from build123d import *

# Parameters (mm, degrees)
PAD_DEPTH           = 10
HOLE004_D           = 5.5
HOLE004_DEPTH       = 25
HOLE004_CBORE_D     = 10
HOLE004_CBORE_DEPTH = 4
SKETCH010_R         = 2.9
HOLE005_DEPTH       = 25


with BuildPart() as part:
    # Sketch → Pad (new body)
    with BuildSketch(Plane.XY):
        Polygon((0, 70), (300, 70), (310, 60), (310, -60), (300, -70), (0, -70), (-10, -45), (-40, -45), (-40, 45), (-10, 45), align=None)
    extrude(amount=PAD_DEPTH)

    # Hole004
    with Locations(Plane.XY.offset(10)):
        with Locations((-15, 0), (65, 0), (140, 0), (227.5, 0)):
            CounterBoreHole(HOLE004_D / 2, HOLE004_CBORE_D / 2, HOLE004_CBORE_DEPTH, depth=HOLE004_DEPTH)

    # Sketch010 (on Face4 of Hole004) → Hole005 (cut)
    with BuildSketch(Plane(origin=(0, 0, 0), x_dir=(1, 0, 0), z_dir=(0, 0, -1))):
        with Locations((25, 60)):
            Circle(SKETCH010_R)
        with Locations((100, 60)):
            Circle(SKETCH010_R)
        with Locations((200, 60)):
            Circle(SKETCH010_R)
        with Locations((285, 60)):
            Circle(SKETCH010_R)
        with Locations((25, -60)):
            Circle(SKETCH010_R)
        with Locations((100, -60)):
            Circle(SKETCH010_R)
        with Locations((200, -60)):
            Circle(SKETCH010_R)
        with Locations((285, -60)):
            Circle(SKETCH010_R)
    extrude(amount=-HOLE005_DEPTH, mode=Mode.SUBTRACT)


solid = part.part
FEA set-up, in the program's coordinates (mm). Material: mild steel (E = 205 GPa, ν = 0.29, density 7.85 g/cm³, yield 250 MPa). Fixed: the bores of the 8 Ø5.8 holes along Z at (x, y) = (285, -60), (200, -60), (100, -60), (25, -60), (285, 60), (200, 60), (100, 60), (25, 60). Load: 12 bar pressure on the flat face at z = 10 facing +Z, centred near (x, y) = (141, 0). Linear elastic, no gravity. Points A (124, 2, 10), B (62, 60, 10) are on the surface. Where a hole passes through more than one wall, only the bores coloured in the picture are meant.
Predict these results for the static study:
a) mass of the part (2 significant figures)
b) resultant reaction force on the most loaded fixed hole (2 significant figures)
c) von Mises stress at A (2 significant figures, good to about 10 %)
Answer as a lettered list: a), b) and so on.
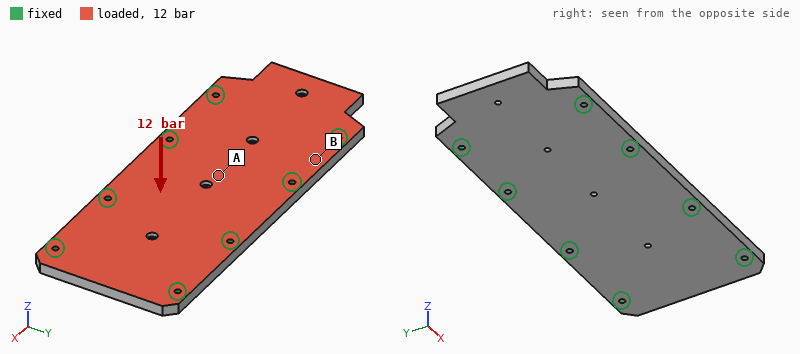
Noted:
a) 3.7 kg
b) 8.0 kN
c) 54 MPa
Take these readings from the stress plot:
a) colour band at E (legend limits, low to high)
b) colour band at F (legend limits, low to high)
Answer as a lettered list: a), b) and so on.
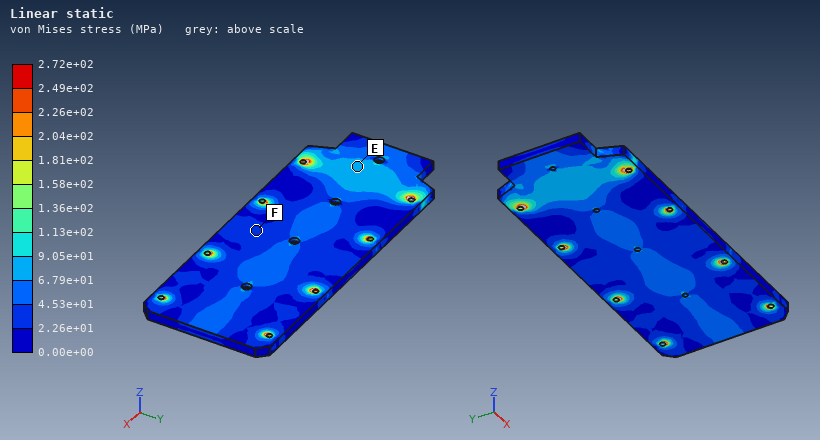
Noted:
a) 6.79e+01 to 9.05e+01 MPa
b) 2.26e+01 to 4.53e+01 MPa
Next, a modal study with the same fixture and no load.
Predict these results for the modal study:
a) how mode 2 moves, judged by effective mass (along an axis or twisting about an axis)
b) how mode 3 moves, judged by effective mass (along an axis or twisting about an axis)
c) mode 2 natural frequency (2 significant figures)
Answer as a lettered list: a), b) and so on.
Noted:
a) along Z
b) twisting about Y
c) 2600 Hz
